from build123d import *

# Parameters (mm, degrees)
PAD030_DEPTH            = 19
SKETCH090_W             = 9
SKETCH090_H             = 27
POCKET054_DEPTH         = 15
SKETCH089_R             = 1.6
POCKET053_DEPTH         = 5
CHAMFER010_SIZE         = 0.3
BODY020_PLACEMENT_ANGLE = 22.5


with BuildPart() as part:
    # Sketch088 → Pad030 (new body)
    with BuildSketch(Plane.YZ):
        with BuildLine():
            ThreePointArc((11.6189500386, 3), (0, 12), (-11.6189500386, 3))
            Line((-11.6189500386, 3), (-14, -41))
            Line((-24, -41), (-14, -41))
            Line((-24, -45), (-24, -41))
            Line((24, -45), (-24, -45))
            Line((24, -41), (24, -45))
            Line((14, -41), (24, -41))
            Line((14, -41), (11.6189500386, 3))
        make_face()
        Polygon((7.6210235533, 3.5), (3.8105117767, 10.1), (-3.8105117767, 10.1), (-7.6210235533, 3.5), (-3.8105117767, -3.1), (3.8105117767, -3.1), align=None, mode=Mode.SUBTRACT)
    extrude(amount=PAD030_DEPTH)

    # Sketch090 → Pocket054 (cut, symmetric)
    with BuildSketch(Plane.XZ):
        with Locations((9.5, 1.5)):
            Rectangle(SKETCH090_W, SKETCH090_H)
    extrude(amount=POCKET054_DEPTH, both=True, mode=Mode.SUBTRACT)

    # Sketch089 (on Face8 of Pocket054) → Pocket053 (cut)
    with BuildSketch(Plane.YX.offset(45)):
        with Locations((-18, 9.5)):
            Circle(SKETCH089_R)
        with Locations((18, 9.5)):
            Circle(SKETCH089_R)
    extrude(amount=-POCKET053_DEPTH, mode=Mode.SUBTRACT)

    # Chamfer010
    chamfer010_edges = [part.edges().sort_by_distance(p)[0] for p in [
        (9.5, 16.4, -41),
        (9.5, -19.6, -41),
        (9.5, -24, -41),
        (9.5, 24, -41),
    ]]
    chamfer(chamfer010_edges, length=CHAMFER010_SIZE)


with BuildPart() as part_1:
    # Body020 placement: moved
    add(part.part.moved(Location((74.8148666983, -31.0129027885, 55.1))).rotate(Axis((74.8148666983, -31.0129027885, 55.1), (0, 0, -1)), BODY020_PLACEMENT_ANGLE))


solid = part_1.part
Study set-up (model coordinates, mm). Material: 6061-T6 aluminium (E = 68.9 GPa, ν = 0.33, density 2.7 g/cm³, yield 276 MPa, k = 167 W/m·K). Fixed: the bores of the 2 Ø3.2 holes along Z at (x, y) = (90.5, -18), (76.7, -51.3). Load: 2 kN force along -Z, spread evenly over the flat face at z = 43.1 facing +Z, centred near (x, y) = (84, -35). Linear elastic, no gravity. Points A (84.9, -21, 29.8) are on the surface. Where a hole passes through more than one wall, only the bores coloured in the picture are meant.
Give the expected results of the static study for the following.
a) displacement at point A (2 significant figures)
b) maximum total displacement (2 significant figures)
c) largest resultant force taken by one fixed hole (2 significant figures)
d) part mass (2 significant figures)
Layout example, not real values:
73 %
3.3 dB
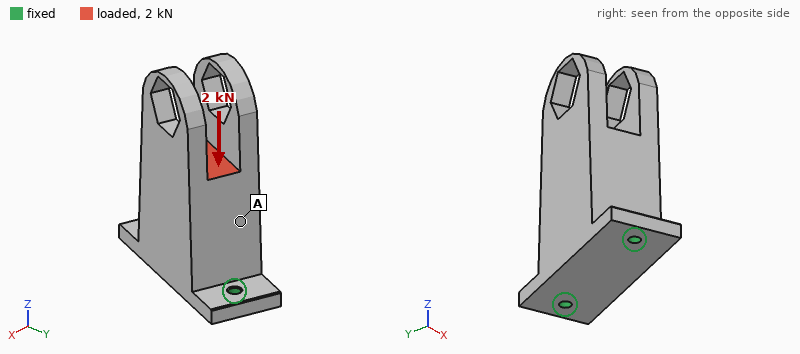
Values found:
10 µm
12 µm
1.1 kN
59 g
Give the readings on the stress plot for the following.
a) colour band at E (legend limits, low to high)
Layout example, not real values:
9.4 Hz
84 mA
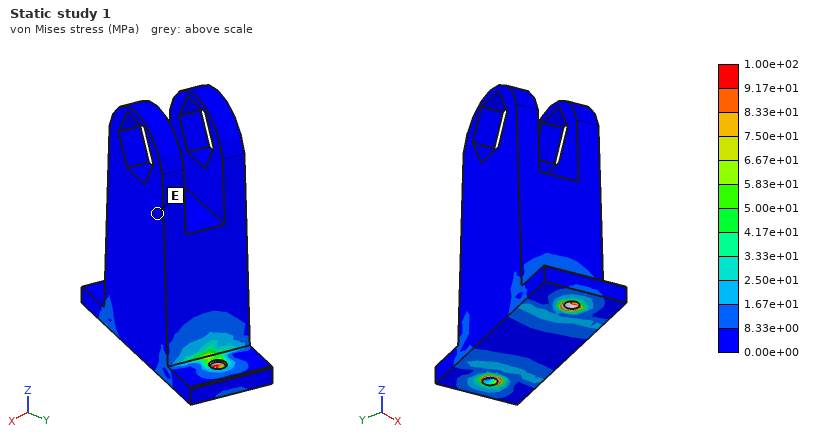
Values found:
0.00e+00 to 8.33e+00 MPa
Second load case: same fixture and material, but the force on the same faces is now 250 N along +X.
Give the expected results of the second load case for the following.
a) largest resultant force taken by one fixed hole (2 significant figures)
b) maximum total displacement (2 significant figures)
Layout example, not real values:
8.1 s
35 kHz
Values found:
160 N
0.12 mm
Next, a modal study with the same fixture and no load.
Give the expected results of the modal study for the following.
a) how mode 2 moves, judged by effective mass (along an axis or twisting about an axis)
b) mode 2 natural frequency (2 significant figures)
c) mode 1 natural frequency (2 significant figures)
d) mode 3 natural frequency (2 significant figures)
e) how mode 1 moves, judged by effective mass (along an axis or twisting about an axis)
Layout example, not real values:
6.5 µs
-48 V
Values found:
along Y
5800 Hz
1700 Hz
8700 Hz
along X
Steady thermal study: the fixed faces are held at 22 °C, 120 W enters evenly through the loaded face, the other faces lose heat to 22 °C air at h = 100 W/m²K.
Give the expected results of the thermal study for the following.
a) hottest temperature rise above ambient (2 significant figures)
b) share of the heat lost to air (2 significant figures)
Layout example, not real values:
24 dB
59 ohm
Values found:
73 K
26 %
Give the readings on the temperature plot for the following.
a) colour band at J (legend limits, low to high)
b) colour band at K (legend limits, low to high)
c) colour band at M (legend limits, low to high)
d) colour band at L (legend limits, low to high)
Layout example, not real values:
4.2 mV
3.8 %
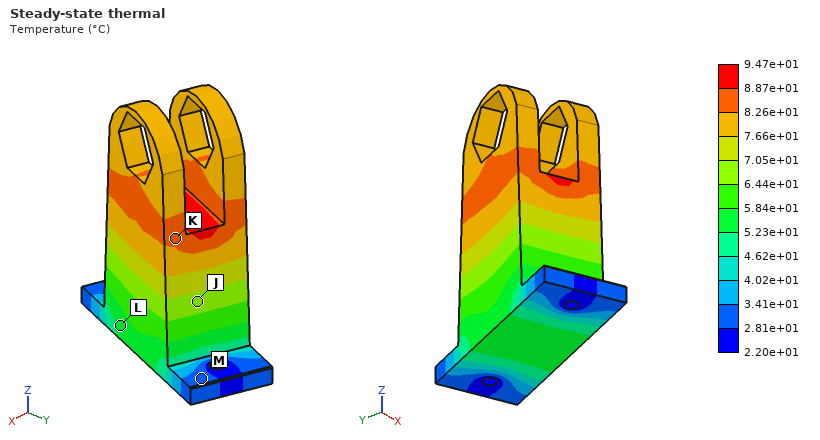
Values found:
6.44e+01 to 7.05e+01 °C
8.26e+01 to 8.87e+01 °C
2.81e+01 to 3.41e+01 °C
5.23e+01 to 5.84e+01 °C
